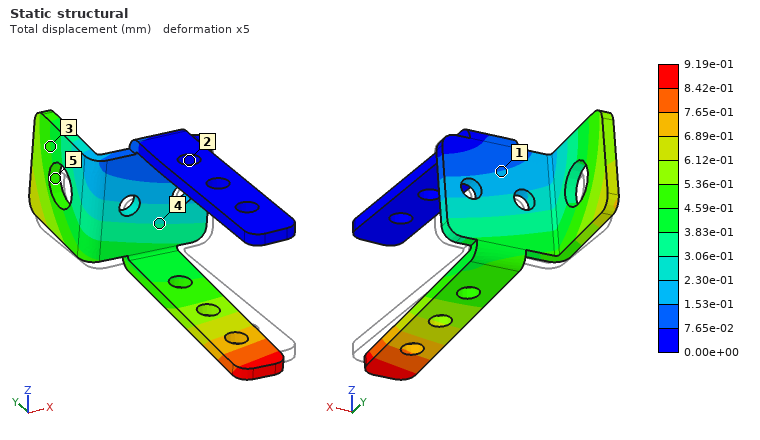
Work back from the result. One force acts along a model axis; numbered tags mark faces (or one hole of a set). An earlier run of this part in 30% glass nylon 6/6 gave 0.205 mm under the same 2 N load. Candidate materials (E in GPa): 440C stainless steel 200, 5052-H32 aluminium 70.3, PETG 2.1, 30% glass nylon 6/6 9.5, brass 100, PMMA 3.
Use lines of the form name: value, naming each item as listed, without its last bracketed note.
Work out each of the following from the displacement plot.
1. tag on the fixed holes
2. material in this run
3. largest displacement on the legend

tag on the fixed holes: 2
material in this run: PETG
largest displacement on the legend: 9.19e-01 mm
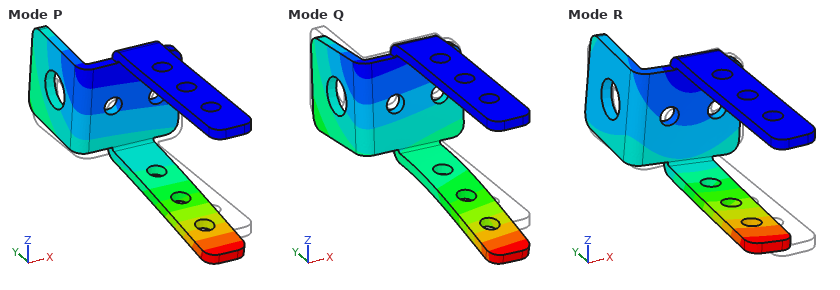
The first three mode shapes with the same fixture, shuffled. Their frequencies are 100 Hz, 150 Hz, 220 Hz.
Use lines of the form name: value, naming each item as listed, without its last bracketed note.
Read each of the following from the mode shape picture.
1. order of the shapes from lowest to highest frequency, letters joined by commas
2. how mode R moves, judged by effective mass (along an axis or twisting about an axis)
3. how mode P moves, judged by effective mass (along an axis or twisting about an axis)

order of the shapes from lowest to highest frequency, letters joined by commas: P, R, Q
how mode R moves, judged by effective mass: along X
how mode P moves, judged by effective mass: along Y
